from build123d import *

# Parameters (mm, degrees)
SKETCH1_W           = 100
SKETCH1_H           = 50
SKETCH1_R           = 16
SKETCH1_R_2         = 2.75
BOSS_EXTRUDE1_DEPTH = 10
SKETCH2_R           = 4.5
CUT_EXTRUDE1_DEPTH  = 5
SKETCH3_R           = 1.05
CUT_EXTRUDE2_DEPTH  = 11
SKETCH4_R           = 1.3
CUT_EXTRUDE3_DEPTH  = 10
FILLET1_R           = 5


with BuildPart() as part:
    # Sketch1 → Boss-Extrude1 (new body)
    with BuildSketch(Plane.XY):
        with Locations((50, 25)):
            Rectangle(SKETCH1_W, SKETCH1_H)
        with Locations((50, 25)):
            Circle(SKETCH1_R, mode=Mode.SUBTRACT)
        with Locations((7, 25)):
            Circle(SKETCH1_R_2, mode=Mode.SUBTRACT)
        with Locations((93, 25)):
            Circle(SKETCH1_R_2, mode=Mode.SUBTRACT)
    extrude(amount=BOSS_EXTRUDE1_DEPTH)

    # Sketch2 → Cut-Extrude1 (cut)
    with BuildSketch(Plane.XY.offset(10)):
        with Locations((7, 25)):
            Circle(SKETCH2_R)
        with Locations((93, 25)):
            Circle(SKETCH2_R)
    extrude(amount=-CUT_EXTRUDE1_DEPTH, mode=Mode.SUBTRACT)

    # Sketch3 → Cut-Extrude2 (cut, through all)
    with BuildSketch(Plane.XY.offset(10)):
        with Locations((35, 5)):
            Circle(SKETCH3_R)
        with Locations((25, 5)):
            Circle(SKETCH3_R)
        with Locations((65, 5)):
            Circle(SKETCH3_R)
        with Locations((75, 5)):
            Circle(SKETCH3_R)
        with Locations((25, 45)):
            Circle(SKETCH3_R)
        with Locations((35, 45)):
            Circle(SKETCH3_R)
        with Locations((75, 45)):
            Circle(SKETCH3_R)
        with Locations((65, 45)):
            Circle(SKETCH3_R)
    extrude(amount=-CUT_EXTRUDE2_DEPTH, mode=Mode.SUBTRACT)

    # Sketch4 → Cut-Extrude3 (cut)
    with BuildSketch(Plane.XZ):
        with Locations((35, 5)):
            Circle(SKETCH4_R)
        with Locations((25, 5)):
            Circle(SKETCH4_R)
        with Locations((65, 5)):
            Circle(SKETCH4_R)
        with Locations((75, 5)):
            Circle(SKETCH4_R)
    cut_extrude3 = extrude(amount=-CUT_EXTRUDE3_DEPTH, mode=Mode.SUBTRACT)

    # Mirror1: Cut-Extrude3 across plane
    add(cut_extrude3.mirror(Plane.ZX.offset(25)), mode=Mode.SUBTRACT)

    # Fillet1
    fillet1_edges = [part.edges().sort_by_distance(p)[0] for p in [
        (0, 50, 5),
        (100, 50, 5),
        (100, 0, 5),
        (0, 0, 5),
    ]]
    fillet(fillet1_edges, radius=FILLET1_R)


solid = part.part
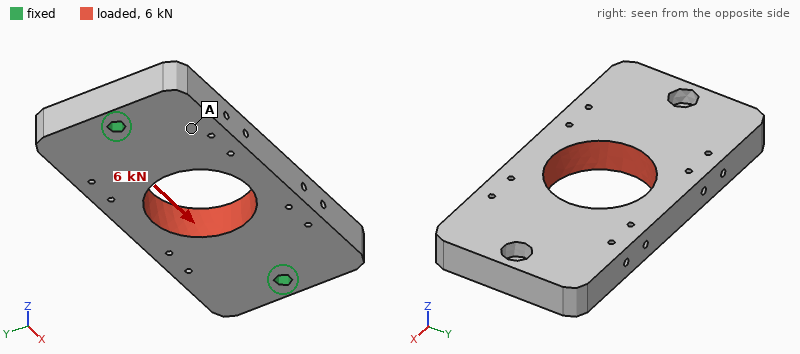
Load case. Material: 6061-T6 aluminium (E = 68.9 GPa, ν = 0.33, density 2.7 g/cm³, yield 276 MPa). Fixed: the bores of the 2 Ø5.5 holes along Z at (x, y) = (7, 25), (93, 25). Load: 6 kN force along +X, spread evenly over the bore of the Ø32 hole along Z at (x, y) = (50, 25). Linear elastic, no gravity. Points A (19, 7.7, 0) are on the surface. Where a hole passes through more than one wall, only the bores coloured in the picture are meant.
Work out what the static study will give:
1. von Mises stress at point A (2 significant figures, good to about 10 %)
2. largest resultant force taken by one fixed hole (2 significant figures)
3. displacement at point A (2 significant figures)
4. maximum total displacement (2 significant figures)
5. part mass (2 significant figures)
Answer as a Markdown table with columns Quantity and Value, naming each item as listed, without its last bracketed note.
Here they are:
| Quantity | Value |
|---|---|
| von Mises stress at point A | 7.8 MPa |
| largest resultant force taken by one fixed hole | 3.0 kN |
| displacement at point A | 6.3 µm |
| maximum total displacement | 10 µm |
| part mass | 110 g |
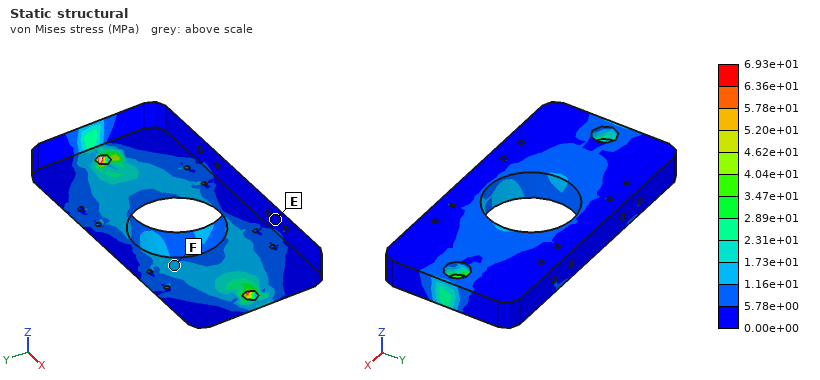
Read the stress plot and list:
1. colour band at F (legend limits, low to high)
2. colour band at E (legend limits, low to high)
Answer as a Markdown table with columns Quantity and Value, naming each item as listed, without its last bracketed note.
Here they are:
| Quantity | Value |
|---|---|
| colour band at F | 1.16e+01 to 1.73e+01 MPa |
| colour band at E | 0.00e+00 to 5.78e+00 MPa |
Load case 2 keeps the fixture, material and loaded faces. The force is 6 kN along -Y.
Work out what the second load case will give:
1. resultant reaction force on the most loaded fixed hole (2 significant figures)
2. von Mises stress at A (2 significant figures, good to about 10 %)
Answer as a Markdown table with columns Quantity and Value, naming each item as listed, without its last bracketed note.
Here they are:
| Quantity | Value |
|---|---|
| resultant reaction force on the most loaded fixed hole | 3.0 kN |
| von Mises stress at A | 10 MPa |
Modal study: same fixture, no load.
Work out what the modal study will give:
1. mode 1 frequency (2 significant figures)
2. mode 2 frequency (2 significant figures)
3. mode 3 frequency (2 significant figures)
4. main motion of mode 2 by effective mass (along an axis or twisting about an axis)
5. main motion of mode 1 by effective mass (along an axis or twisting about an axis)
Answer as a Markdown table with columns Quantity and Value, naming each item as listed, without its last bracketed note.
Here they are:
| Quantity | Value |
|---|---|
| mode 1 frequency | 3600 Hz |
| mode 2 frequency | 4200 Hz |
| mode 3 frequency | 6900 Hz |
| main motion of mode 2 by effective mass | along Z |
| main motion of mode 1 by effective mass | twisting about X |
